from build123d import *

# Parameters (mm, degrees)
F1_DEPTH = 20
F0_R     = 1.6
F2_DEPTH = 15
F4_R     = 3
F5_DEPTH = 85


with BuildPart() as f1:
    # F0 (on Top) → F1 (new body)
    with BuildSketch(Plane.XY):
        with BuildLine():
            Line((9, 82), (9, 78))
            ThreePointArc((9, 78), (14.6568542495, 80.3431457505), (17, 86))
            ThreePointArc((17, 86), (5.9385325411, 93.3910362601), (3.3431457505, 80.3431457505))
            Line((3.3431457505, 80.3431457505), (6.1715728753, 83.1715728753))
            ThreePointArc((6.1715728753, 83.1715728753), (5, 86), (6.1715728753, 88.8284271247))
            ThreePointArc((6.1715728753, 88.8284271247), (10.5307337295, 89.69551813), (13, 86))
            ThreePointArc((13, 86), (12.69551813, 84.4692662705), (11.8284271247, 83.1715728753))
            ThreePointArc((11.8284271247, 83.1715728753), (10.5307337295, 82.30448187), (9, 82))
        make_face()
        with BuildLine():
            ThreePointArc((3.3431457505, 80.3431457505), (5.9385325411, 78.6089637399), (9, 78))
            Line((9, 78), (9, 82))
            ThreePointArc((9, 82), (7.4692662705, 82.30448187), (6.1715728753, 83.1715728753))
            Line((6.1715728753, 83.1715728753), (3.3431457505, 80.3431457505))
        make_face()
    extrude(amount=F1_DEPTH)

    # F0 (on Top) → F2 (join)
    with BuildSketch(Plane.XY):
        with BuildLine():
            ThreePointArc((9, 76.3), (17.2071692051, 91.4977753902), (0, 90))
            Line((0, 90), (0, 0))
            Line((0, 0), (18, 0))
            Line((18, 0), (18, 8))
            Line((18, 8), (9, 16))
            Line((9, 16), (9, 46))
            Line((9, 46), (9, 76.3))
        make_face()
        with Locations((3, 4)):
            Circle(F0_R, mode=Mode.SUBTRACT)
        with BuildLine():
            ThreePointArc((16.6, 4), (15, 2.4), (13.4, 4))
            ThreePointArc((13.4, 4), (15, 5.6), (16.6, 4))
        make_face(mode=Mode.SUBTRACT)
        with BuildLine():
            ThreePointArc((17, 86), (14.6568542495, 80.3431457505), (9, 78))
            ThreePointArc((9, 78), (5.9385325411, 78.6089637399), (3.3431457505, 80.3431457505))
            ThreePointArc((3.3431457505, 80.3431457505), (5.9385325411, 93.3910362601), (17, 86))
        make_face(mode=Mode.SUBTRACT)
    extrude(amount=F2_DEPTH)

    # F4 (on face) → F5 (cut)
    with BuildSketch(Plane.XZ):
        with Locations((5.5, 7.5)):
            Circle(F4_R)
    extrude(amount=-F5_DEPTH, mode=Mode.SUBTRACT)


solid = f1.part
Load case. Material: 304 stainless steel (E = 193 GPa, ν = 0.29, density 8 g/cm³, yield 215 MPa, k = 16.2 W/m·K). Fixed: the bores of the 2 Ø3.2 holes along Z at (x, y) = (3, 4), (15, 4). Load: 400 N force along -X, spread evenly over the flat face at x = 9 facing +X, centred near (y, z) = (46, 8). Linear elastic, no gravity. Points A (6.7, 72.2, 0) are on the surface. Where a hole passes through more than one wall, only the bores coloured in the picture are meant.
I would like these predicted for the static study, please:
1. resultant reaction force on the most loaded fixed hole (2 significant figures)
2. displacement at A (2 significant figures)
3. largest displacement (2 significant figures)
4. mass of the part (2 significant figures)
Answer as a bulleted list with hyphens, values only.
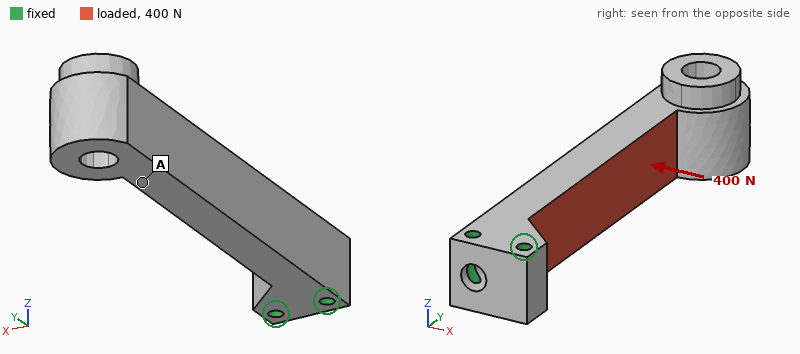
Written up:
- 1.4 kN
- 0.092 mm
- 0.14 mm
- 110 g
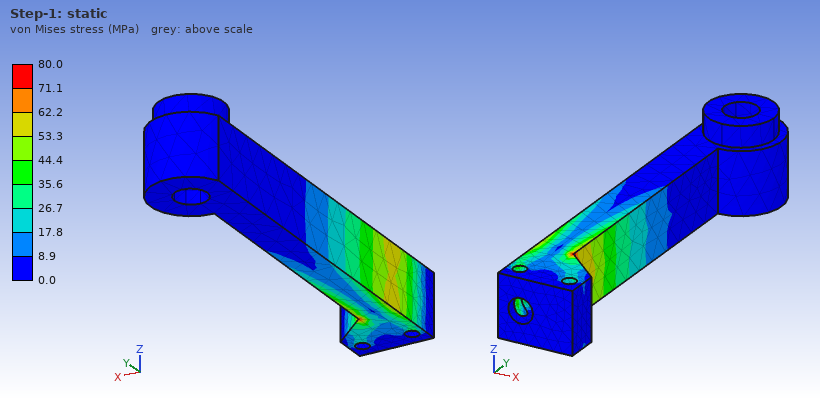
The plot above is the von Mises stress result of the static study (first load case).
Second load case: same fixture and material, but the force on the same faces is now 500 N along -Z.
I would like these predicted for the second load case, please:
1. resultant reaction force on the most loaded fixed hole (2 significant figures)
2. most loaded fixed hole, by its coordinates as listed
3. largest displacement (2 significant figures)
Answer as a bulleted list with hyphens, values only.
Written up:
- 370 N
- (15, 4)
- 85 µm
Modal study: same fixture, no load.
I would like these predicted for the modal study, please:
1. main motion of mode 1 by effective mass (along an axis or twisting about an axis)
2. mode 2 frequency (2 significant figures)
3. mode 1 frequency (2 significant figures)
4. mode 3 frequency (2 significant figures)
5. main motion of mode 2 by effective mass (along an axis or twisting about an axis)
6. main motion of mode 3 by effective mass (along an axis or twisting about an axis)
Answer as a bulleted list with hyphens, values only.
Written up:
- along X
- 1200 Hz
- 780 Hz
- 4300 Hz
- along Z
- twisting about Y
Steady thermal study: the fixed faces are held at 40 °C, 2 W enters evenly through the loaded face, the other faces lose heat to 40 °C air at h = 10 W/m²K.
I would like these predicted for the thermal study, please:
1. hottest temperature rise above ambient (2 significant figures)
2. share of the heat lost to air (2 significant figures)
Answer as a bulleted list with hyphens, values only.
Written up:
- 20 K
- 44 %
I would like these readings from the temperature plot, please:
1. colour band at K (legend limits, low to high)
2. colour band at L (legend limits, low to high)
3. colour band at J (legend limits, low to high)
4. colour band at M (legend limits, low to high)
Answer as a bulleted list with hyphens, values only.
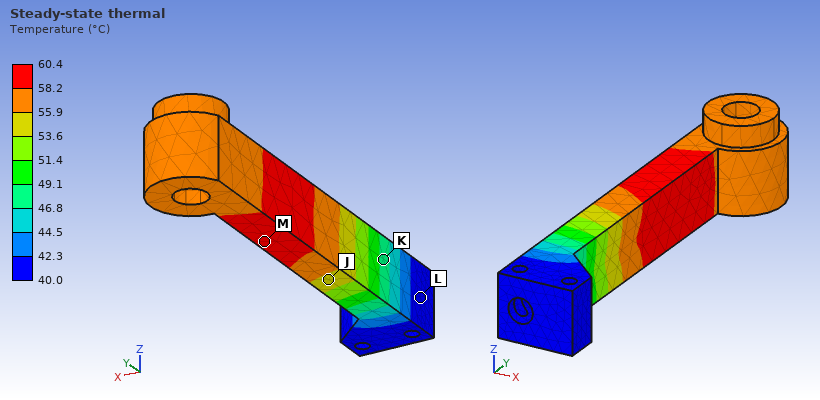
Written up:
- 46.8 to 49.1 °C
- 40.0 to 42.3 °C
- 53.6 to 55.9 °C
- 58.2 to 60.4 °C
